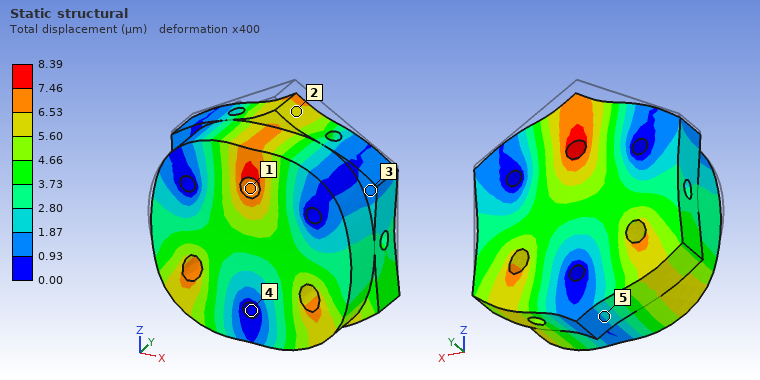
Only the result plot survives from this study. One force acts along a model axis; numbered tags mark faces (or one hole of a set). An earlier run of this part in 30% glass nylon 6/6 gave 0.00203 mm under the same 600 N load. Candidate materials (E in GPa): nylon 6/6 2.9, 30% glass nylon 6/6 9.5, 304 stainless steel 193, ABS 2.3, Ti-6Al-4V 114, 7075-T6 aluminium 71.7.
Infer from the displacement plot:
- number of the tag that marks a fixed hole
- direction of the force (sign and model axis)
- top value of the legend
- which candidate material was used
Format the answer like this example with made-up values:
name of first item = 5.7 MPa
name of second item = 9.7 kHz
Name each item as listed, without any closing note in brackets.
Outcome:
number of the tag that marks a fixed hole = 4
direction of the force = -Z
top value of the legend = 8.39 µm
which candidate material was used = ABS
